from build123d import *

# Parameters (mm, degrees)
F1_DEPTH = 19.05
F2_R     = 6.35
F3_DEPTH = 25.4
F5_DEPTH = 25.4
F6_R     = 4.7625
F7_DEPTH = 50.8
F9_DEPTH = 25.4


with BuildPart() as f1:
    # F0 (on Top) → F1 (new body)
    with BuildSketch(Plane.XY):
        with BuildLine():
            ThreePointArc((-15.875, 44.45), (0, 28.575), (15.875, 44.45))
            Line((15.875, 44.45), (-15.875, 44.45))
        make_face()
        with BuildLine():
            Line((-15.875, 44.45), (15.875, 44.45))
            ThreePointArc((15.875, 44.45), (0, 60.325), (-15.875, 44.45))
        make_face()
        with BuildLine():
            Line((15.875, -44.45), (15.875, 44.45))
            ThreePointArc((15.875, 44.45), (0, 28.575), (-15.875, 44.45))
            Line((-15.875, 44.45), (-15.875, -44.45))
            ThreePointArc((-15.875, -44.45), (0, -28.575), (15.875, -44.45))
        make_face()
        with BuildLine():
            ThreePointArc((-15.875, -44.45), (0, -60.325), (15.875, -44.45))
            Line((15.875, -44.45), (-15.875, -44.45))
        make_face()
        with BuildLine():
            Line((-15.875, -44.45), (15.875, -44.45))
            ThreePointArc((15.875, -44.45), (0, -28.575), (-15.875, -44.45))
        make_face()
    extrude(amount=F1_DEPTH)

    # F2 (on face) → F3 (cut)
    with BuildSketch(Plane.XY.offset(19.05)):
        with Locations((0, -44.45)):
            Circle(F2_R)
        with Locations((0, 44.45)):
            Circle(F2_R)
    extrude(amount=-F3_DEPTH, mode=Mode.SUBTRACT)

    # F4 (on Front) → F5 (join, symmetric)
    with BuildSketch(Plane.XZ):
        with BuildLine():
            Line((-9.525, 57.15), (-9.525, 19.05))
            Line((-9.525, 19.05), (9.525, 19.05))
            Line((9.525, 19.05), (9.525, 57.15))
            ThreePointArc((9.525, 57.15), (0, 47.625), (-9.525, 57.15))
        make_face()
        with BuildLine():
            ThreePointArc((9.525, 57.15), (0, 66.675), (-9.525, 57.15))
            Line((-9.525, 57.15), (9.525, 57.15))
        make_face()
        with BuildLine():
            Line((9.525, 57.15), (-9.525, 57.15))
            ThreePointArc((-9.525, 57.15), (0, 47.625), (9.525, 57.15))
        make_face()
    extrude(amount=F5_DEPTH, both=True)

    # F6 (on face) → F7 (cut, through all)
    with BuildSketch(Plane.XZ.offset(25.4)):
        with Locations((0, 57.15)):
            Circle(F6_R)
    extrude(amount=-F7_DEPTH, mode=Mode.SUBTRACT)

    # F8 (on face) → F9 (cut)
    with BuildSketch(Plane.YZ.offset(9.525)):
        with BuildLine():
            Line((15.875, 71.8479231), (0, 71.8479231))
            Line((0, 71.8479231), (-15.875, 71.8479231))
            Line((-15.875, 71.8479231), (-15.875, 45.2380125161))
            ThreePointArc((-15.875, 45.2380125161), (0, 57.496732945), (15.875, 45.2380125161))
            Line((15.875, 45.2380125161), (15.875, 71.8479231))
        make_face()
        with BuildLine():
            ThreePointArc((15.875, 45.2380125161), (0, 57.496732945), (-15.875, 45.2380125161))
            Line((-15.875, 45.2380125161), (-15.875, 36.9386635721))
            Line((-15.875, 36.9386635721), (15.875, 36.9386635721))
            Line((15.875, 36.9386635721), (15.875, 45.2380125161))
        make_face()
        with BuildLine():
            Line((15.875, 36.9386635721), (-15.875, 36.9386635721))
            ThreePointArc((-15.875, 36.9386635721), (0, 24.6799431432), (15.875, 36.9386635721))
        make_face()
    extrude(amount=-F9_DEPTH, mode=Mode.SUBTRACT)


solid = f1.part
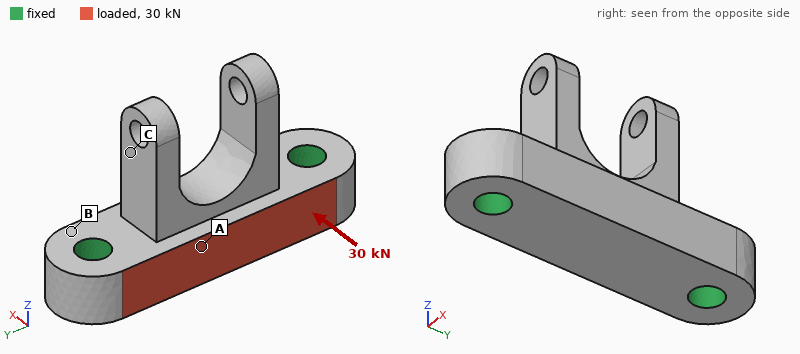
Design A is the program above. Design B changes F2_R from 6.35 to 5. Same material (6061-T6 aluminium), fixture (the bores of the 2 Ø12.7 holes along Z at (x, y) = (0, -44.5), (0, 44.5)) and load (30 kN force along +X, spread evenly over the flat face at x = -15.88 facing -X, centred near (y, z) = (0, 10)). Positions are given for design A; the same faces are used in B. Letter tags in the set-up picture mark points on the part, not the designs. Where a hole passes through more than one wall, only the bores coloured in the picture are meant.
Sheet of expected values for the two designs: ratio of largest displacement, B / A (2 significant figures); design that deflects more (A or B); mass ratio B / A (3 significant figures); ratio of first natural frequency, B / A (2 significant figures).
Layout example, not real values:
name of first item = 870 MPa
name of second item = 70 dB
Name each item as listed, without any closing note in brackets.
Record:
ratio of largest displacement, B / A = 1.2
design that deflects more = B
mass ratio B / A = 1.02
ratio of first natural frequency, B / A = 0.96
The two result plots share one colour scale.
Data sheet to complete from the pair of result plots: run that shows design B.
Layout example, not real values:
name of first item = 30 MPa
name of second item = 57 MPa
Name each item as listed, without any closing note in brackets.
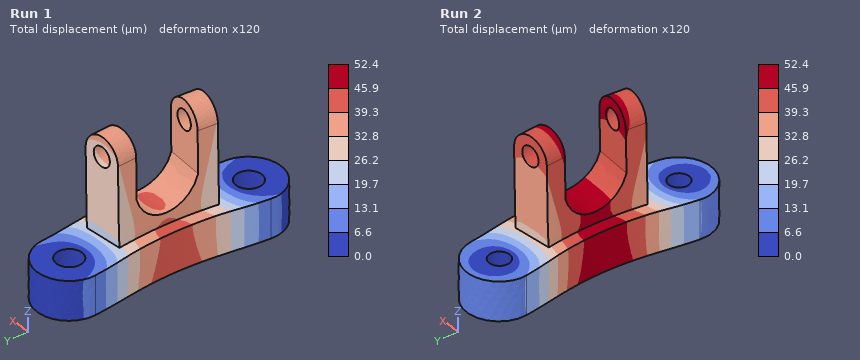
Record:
run that shows design B = Run 2
